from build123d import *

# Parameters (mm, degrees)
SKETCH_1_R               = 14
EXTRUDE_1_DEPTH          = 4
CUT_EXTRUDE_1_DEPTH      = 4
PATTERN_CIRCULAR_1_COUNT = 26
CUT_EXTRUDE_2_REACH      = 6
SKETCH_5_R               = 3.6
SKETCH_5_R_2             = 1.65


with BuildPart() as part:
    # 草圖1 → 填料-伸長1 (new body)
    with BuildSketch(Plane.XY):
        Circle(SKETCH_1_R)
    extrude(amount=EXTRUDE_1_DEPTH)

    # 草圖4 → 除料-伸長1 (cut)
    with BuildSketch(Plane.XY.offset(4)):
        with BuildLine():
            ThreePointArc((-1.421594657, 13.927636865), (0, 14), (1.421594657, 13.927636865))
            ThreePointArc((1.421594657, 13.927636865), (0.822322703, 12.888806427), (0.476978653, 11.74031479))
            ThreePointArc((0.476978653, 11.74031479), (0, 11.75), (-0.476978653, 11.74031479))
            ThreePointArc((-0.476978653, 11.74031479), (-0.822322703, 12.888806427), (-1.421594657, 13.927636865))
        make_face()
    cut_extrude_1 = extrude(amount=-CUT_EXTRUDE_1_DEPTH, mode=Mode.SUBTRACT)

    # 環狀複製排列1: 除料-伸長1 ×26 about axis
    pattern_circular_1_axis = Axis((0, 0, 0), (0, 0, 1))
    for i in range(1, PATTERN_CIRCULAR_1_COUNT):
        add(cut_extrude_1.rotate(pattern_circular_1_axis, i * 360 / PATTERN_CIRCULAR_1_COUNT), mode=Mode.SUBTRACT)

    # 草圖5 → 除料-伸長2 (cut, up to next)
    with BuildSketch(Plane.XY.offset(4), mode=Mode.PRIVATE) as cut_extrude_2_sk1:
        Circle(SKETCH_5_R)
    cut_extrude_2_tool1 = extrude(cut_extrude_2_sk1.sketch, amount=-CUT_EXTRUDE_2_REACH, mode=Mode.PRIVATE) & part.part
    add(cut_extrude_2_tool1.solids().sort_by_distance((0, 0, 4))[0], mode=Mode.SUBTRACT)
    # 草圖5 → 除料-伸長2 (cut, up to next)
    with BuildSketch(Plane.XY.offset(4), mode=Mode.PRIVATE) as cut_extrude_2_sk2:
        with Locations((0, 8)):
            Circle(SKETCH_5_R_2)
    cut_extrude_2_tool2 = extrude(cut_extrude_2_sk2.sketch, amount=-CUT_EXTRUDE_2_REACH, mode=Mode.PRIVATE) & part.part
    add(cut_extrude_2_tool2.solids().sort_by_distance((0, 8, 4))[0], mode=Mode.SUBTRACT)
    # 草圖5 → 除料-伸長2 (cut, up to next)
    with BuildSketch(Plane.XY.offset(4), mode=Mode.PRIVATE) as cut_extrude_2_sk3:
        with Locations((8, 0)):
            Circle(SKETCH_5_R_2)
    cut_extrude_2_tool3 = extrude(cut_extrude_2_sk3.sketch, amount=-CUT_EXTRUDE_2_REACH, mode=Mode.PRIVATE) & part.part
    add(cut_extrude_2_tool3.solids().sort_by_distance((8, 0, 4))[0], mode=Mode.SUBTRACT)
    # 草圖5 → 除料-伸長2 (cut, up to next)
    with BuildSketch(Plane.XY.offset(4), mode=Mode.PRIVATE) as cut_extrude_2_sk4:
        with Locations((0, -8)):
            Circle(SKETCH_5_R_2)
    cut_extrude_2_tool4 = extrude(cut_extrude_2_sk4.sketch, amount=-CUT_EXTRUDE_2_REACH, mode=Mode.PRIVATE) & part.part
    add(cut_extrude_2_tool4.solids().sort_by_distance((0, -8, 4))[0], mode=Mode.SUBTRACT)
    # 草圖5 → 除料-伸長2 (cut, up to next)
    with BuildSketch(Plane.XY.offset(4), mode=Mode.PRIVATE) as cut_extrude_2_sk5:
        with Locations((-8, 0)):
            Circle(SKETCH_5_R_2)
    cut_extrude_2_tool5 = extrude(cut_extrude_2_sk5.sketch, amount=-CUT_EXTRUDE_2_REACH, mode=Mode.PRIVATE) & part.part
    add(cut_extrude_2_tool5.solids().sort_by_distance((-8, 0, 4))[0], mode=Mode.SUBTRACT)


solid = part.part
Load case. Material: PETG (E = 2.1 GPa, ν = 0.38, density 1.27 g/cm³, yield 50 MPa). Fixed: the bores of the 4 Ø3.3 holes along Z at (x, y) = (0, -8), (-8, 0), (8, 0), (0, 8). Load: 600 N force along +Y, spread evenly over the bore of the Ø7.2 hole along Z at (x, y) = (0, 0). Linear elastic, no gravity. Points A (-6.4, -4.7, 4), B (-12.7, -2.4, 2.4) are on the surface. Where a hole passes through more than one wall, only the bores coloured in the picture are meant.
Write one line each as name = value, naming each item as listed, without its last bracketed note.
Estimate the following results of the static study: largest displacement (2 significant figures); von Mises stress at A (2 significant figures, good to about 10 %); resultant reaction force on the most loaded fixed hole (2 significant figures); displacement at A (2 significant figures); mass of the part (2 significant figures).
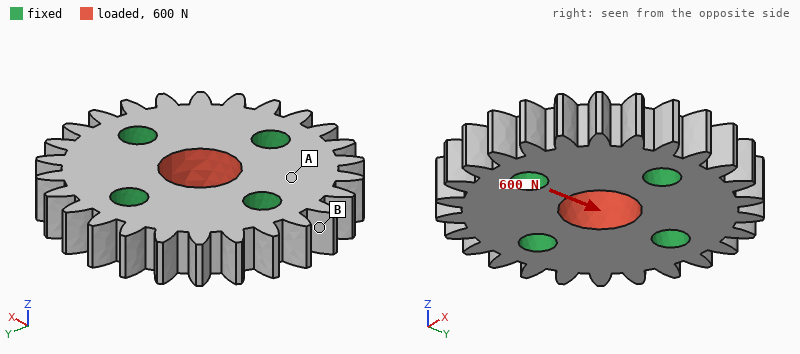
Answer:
largest displacement = 20 µm
von Mises stress at A = 2.4 MPa
resultant reaction force on the most loaded fixed hole = 190 N
displacement at A = 7.7 µm
mass of the part = 2.2 g
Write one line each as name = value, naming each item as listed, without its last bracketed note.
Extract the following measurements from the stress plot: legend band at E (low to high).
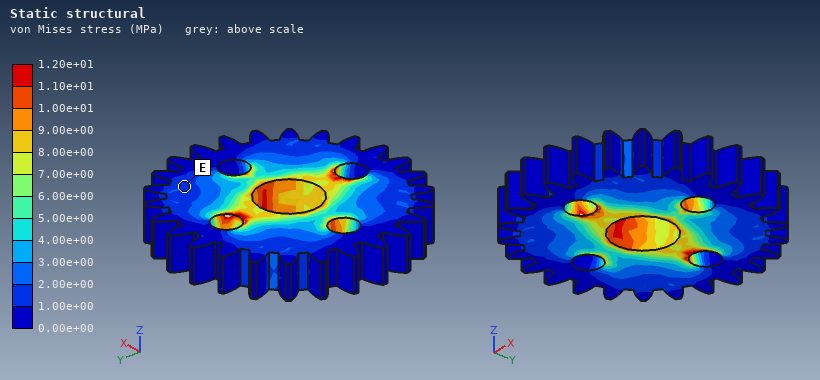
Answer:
legend band at E = 1.00e+00 to 2.00e+00 MPa
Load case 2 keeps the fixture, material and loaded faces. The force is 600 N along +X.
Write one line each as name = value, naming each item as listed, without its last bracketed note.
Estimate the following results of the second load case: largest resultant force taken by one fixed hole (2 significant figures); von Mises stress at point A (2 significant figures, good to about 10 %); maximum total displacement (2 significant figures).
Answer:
largest resultant force taken by one fixed hole = 190 N
von Mises stress at point A = 2.4 MPa
maximum total displacement = 20 µm
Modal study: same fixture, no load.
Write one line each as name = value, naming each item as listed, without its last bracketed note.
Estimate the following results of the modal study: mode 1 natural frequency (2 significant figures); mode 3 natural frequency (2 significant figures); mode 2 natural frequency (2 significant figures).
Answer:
mode 1 natural frequency = 15 kHz
mode 3 natural frequency = 16 kHz
mode 2 natural frequency = 16 kHz
